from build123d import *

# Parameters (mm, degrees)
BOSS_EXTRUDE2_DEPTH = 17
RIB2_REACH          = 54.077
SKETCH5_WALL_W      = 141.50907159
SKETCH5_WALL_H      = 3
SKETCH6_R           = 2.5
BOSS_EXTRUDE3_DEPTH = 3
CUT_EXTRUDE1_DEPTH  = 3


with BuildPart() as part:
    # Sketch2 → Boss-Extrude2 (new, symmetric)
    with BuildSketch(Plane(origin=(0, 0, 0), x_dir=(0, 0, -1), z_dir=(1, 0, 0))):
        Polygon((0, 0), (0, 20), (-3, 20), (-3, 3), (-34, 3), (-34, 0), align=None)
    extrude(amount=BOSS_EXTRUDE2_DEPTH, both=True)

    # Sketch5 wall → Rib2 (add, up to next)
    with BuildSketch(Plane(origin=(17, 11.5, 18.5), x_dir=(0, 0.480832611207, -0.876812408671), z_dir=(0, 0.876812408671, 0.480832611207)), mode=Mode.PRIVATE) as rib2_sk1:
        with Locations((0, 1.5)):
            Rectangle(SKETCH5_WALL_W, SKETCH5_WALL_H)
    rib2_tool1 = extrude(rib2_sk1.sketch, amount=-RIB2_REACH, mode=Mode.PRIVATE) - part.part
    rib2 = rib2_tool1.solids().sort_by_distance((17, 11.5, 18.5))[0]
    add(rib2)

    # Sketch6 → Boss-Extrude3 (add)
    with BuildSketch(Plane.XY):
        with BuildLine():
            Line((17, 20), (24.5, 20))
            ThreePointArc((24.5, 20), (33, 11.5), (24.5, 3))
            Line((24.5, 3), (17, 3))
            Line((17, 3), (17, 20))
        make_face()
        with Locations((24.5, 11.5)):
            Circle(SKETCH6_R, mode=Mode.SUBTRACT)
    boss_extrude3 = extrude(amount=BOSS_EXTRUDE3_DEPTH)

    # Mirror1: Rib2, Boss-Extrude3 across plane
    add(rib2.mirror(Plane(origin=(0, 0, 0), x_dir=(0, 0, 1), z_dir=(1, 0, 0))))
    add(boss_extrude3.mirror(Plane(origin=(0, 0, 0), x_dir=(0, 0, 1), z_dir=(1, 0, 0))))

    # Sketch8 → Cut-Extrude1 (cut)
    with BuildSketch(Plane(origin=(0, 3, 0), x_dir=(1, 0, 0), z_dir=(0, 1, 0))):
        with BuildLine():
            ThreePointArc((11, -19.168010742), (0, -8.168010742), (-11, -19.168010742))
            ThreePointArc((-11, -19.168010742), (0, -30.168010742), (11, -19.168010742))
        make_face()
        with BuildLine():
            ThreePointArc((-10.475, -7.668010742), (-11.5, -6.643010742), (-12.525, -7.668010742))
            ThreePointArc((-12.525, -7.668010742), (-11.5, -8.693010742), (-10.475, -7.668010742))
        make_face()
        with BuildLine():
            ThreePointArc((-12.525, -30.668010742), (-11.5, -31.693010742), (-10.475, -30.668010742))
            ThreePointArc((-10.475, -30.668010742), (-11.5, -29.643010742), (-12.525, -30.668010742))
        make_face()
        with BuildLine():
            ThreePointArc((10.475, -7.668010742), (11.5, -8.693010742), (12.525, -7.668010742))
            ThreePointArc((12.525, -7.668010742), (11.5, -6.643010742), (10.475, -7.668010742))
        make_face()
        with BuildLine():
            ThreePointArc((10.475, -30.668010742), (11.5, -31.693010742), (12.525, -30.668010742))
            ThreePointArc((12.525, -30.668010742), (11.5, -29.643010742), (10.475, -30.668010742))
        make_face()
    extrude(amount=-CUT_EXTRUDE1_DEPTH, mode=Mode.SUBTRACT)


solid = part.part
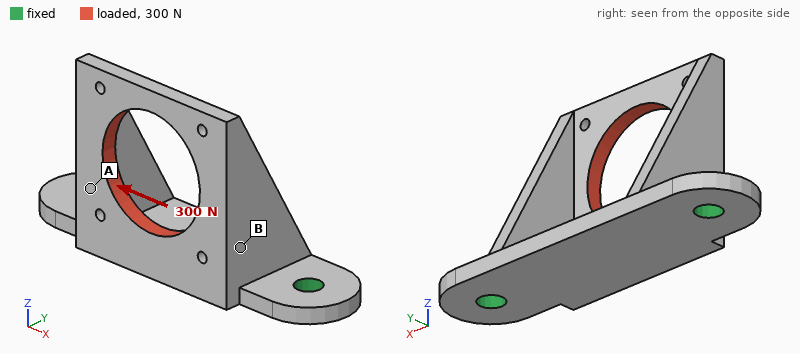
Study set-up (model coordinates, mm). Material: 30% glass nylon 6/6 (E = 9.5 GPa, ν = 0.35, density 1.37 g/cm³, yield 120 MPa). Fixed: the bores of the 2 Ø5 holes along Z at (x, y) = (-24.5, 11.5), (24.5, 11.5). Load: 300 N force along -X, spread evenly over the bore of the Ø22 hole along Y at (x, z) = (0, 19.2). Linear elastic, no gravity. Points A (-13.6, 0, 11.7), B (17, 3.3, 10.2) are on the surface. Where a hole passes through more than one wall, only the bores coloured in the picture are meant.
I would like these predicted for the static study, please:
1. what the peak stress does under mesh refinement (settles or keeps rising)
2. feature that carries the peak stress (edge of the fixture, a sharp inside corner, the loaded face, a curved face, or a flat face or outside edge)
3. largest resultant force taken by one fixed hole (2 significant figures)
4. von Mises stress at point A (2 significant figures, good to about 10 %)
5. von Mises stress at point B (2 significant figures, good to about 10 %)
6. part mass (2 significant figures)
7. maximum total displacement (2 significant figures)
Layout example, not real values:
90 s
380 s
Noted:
keeps rising
edge of the fixture
210 N
5.6 MPa
11 MPa
9.5 g
0.30 mm
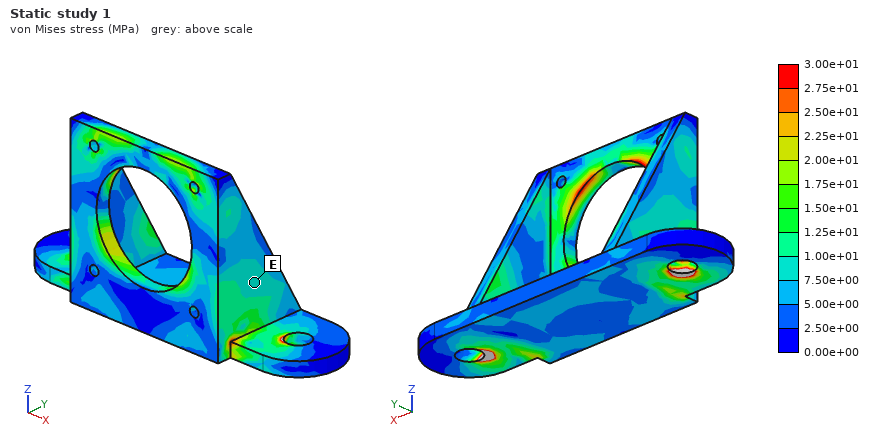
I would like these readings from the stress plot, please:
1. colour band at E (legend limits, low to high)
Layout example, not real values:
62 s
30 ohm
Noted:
7.50e+00 to 1.00e+01 MPa
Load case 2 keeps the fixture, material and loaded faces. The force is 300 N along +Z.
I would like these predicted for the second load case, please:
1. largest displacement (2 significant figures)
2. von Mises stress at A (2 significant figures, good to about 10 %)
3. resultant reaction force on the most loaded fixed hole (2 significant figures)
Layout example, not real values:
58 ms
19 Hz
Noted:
0.53 mm
5.2 MPa
160 N
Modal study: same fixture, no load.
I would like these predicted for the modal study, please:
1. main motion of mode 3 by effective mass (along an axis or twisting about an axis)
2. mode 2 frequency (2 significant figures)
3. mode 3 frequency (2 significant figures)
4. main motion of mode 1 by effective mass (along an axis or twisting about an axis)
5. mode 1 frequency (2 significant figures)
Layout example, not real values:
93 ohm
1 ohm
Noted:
along Z
2600 Hz
4200 Hz
along Y
1600 Hz
